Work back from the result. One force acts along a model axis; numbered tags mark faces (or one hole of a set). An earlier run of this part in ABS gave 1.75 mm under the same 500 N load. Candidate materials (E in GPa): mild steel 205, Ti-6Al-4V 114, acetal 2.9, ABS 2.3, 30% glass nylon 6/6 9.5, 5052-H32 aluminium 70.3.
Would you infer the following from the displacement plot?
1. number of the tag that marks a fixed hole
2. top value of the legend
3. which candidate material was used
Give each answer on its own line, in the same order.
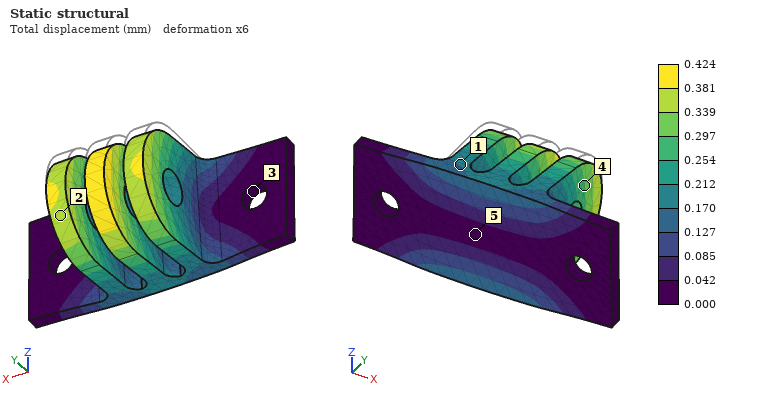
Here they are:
3
0.424 mm
30% glass nylon 6/6
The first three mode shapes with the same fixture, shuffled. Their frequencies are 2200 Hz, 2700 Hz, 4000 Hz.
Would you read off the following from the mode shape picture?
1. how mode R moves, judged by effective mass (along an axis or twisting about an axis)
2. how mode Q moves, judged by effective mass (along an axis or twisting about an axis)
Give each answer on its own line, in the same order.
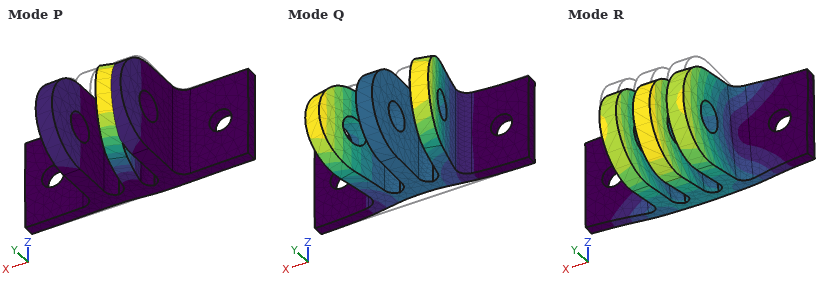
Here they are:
along Z
along Y
